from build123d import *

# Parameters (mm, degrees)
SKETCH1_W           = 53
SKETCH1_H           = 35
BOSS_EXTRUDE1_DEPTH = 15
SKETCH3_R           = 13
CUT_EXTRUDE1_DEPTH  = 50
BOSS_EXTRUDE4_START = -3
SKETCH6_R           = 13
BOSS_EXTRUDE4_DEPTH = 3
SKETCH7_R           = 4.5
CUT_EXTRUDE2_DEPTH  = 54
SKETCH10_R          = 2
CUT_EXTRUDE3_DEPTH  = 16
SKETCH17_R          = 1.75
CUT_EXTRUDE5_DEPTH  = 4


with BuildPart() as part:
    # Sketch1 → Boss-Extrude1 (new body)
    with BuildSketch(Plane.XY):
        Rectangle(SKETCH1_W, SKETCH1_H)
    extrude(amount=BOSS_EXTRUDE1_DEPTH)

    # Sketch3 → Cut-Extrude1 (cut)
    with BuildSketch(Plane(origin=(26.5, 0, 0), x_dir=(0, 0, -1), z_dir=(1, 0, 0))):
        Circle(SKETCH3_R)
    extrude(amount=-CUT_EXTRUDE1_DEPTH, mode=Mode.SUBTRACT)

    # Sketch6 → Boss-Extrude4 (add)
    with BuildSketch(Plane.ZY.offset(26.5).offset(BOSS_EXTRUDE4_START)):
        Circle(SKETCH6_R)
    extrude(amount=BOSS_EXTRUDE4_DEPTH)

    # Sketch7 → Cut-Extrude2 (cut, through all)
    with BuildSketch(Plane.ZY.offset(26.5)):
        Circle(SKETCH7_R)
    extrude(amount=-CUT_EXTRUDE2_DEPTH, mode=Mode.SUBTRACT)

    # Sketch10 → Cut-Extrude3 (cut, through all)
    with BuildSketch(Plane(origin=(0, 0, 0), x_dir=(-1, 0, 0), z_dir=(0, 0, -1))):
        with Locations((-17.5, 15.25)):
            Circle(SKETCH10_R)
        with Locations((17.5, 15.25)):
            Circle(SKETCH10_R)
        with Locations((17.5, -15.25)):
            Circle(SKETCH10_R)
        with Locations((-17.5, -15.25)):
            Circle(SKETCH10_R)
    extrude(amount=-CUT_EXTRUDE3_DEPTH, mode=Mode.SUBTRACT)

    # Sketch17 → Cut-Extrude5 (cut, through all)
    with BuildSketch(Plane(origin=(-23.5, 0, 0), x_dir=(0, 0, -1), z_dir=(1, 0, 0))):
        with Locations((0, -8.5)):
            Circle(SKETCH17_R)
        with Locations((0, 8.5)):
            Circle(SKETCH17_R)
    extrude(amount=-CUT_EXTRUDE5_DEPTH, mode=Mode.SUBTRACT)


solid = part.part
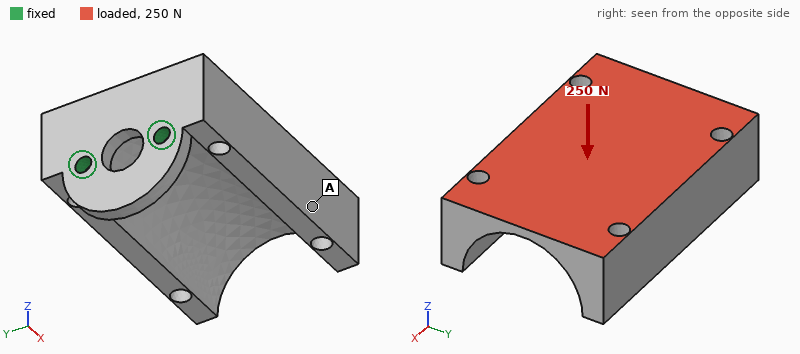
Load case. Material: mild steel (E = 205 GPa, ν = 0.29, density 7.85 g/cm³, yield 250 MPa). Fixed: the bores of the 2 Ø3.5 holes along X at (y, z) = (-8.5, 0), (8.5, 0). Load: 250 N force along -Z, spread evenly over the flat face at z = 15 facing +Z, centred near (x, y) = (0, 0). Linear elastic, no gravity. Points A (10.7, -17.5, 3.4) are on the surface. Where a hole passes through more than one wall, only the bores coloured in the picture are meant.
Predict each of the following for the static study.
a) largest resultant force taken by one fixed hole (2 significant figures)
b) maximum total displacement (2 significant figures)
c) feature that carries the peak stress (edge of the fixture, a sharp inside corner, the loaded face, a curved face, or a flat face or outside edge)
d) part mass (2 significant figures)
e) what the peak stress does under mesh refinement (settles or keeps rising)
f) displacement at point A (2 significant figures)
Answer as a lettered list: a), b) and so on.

a) 130 N
b) 0.13 mm
c) edge of the fixture
d) 110 g
e) keeps rising
f) 0.086 mm
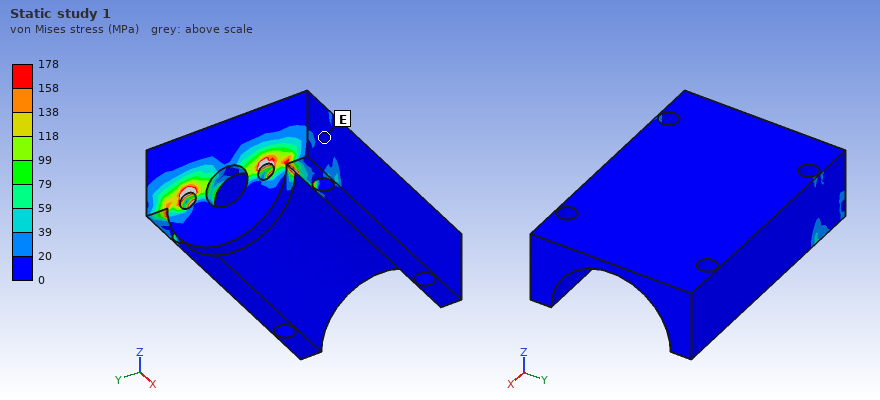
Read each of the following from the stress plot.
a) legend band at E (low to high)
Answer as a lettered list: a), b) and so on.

a) 0 to 20 MPa
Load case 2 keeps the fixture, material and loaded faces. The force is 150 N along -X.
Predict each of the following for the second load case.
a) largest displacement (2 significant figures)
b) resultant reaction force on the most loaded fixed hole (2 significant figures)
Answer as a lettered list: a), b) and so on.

a) 37 µm
b) 75 N
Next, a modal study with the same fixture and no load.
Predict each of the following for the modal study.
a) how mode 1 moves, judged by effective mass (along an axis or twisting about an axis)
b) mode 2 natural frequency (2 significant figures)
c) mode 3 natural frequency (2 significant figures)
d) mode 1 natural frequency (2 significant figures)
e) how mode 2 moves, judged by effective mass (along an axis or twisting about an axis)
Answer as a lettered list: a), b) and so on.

a) along Z
b) 1800 Hz
c) 4500 Hz
d) 840 Hz
e) along Y
